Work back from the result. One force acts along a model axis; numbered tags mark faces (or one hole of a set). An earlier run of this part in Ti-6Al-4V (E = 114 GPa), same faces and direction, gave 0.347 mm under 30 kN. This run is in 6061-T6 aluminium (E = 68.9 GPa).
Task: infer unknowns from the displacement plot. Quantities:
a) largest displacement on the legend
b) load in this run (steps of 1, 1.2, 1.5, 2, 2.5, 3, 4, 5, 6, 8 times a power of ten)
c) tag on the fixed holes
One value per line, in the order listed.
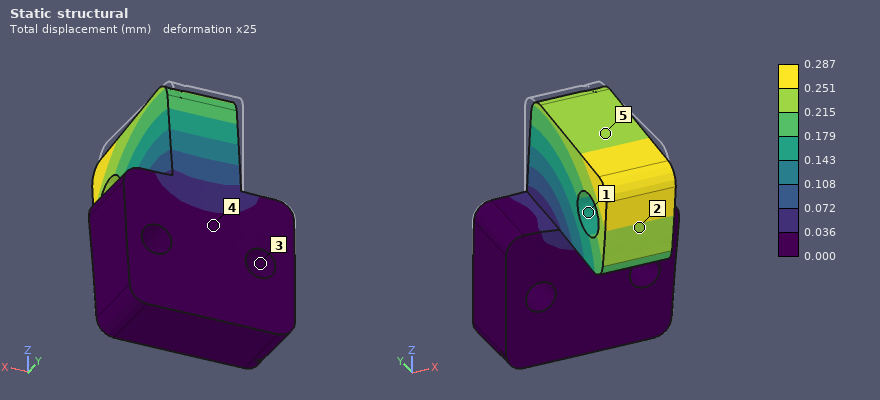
0.287 mm
15 kN
3
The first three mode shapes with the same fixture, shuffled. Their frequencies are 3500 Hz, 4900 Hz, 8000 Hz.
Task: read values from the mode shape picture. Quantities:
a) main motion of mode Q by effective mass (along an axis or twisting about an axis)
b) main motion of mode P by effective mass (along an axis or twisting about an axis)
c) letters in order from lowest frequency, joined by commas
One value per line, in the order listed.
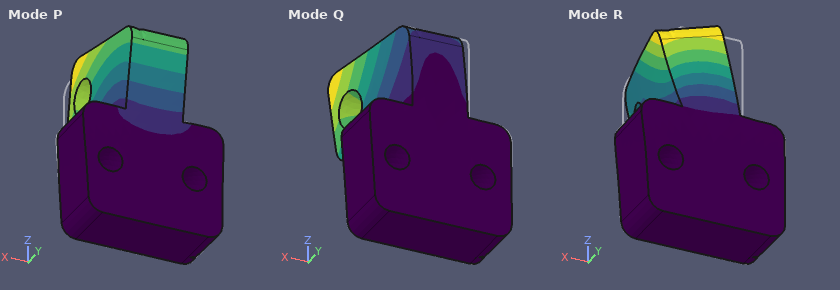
along X
along Y
P, Q, R
